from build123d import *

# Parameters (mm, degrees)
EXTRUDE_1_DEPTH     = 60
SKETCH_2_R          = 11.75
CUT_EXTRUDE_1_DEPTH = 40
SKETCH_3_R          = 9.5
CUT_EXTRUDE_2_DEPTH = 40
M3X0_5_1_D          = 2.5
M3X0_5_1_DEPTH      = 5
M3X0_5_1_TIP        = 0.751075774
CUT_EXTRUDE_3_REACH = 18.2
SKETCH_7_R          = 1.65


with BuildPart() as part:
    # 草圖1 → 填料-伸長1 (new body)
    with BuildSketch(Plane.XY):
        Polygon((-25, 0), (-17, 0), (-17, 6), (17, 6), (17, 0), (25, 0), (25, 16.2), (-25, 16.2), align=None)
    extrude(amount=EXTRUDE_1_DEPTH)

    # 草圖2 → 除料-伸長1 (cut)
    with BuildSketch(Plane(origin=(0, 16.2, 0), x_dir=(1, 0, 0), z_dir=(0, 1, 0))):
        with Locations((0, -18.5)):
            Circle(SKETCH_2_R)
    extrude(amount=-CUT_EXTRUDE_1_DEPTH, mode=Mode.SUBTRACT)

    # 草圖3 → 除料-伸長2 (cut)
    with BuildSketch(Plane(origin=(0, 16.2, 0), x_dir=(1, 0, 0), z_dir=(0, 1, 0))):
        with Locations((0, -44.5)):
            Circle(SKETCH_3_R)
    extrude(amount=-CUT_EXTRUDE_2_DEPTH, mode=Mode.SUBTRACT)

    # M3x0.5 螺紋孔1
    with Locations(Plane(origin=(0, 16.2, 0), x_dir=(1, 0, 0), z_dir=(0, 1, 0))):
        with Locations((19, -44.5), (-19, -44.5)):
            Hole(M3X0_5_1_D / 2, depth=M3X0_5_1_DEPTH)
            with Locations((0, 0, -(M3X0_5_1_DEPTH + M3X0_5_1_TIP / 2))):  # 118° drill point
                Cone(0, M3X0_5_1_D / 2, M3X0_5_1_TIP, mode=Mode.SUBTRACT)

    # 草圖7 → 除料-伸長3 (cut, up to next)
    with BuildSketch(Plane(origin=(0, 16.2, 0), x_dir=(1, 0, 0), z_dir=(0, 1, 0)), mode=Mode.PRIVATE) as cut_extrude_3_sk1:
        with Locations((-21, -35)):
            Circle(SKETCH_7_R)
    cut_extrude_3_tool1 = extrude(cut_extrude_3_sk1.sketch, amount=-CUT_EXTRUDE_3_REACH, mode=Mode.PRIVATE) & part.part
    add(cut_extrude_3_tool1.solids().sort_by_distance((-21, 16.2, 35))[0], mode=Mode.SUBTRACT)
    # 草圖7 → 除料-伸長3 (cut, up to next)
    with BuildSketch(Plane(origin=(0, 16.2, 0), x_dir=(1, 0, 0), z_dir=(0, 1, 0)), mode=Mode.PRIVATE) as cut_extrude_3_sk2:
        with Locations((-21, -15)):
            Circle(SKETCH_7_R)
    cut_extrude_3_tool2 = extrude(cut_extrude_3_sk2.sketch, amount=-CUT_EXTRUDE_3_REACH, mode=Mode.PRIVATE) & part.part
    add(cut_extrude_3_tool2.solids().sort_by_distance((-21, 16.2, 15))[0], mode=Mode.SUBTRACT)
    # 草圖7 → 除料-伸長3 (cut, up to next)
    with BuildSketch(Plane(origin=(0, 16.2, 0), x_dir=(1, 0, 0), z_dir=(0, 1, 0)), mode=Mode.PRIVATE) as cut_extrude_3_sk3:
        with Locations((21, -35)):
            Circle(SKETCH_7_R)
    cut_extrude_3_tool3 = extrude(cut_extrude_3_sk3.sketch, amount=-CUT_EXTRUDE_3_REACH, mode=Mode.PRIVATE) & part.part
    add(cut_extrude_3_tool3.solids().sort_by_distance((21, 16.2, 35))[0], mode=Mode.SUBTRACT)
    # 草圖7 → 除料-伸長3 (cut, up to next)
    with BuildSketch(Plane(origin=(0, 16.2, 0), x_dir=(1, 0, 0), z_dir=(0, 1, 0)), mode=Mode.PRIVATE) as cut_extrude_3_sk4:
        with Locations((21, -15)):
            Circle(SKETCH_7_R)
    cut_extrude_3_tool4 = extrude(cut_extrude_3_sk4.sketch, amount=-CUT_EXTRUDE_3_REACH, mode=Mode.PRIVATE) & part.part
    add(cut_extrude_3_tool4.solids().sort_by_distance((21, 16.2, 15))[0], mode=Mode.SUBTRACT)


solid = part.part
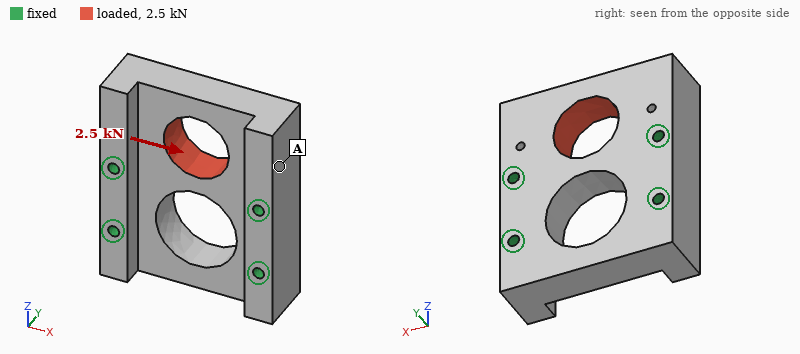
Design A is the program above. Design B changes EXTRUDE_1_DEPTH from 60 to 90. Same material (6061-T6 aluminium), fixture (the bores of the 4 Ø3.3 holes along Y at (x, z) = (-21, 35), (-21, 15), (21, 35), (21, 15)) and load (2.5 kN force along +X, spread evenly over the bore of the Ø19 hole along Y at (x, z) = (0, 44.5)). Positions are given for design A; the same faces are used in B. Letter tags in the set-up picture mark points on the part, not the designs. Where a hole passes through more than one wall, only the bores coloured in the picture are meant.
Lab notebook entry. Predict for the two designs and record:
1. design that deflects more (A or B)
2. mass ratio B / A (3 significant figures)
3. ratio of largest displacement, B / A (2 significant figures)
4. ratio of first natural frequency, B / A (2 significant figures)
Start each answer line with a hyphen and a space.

- A
- 1.64
- 0.73
- 0.26
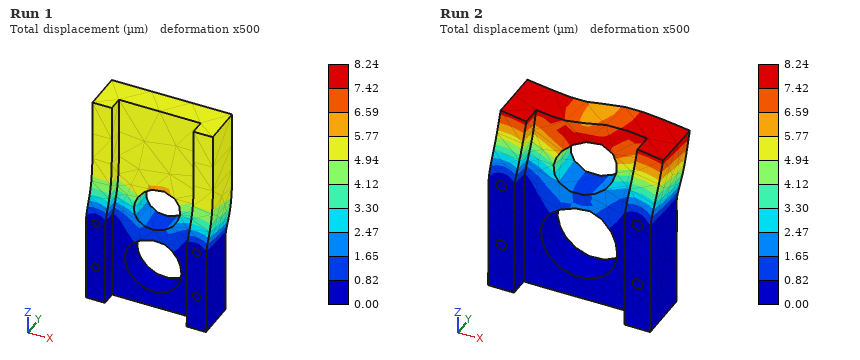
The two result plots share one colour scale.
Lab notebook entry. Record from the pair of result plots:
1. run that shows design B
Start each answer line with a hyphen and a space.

- Run 1
